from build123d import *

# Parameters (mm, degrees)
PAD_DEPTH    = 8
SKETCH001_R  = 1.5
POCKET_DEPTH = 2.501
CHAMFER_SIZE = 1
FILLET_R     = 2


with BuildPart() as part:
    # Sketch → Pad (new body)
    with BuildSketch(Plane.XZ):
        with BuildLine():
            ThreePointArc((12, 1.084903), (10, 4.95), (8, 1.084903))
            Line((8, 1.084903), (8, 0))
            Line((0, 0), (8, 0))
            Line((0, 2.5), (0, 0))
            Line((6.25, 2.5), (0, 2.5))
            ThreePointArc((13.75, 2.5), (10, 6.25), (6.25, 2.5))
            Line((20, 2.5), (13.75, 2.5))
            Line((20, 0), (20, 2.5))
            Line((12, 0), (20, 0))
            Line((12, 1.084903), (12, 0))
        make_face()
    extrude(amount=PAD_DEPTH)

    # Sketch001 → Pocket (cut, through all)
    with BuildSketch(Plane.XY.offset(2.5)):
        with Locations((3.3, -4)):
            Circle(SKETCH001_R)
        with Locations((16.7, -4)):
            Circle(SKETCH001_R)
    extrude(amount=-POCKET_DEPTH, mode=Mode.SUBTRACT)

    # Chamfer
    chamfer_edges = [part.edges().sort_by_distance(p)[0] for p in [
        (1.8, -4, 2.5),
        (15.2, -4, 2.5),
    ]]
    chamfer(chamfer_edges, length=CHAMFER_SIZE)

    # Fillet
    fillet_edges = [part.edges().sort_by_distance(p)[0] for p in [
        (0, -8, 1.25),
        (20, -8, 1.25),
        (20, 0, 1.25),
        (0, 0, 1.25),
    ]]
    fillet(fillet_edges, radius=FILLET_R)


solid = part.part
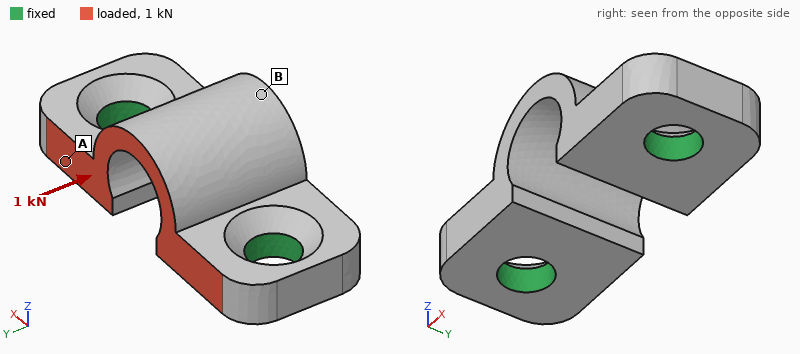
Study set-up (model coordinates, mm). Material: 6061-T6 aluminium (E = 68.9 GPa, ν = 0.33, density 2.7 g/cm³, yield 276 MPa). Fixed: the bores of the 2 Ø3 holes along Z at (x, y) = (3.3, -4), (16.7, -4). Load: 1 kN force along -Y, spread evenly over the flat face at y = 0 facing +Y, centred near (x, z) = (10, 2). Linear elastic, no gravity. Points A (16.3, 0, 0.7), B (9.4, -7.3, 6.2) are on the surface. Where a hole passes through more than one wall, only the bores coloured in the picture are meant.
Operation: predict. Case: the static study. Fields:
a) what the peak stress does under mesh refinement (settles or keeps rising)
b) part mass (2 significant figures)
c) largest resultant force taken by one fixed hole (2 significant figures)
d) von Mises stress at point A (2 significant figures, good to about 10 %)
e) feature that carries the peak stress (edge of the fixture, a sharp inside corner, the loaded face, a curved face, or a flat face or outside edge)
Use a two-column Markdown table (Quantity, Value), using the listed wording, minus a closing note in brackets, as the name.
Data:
| Quantity | Value |
|---|---|
| what the peak stress does under mesh refinement | keeps rising |
| part mass | 0.97 g |
| largest resultant force taken by one fixed hole | 500 N |
| von Mises stress at point A | 47 MPa |
| feature that carries the peak stress | edge of the fixture |
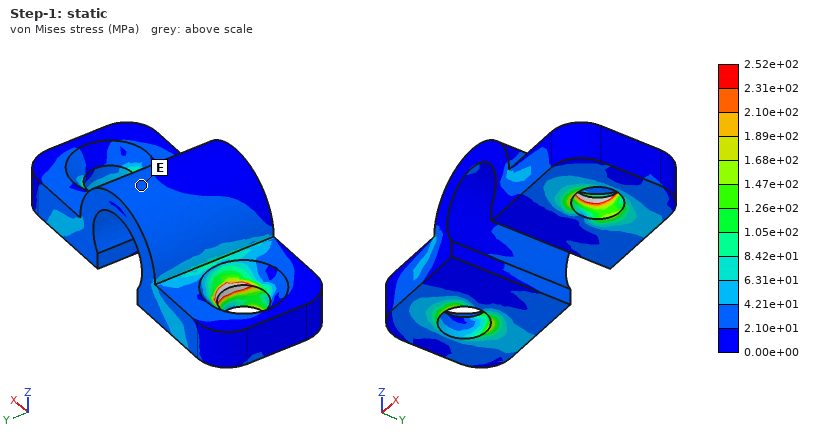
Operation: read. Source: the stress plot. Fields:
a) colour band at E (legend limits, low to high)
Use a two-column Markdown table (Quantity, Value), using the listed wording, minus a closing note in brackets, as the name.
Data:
| Quantity | Value |
|---|---|
| colour band at E | 2.10e+01 to 4.21e+01 MPa |
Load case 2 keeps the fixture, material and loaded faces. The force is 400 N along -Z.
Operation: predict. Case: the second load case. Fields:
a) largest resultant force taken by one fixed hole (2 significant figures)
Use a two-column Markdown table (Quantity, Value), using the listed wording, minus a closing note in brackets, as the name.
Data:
| Quantity | Value |
|---|---|
| largest resultant force taken by one fixed hole | 200 N |
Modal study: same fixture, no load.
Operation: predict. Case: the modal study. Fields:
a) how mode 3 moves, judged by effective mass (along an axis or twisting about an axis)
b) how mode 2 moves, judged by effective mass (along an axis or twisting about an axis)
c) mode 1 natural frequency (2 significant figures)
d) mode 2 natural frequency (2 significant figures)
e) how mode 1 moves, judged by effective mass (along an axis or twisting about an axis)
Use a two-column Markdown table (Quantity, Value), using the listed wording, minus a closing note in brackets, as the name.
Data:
| Quantity | Value |
|---|---|
| how mode 3 moves, judged by effective mass | along Z |
| how mode 2 moves, judged by effective mass | along X |
| mode 1 natural frequency | 40 kHz |
| mode 2 natural frequency | 63 kHz |
| how mode 1 moves, judged by effective mass | along Y |
